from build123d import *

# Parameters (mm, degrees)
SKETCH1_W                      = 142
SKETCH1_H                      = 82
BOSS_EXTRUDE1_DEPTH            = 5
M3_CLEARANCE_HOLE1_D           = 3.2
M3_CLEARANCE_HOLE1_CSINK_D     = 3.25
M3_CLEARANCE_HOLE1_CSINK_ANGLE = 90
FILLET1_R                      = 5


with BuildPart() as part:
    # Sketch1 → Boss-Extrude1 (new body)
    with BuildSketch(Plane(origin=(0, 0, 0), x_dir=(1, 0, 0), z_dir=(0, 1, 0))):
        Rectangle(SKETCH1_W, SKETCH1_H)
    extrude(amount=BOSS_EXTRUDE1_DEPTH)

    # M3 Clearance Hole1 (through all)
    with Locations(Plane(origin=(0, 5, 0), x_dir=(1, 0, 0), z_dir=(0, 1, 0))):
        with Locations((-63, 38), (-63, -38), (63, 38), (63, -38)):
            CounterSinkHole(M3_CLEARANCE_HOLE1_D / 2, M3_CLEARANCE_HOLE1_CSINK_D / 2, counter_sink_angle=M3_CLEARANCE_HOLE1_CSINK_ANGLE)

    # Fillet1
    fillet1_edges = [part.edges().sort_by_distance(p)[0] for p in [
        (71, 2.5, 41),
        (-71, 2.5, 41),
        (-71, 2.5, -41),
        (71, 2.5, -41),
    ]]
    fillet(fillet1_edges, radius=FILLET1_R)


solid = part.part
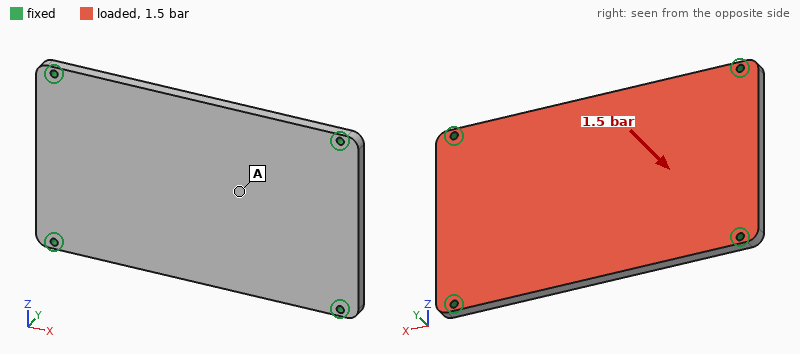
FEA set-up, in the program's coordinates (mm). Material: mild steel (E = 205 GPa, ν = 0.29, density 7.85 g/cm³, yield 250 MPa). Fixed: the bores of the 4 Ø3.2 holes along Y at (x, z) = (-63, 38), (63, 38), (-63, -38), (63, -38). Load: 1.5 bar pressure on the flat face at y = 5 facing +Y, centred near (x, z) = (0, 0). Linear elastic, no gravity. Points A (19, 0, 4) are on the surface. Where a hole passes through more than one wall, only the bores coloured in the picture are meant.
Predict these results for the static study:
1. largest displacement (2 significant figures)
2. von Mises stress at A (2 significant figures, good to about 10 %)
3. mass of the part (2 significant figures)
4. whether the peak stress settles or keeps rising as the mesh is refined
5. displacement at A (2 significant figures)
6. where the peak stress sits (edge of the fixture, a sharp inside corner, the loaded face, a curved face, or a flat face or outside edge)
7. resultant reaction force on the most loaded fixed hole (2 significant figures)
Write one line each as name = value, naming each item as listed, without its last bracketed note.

largest displacement = 83 µm
von Mises stress at A = 23 MPa
mass of the part = 450 g
whether the peak stress settles or keeps rising as the mesh is refined = keeps rising
displacement at A = 74 µm
where the peak stress sits = edge of the fixture
resultant reaction force on the most loaded fixed hole = 430 N
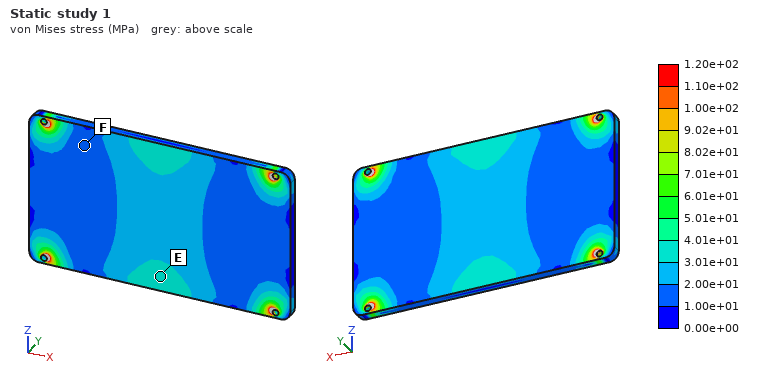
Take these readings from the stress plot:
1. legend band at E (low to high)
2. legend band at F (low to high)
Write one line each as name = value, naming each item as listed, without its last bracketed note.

legend band at E = 3.01e+01 to 4.01e+01 MPa
legend band at F = 1.00e+01 to 2.00e+01 MPa
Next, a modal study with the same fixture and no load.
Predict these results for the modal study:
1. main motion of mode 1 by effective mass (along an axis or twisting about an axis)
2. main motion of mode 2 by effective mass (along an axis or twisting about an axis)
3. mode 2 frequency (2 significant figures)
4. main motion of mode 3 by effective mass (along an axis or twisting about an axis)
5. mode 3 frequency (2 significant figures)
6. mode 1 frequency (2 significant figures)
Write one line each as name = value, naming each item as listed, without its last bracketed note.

main motion of mode 1 by effective mass = along Y
main motion of mode 2 by effective mass = twisting about X
mode 2 frequency = 2200 Hz
main motion of mode 3 by effective mass = twisting about Z
mode 3 frequency = 3200 Hz
mode 1 frequency = 1200 Hz
